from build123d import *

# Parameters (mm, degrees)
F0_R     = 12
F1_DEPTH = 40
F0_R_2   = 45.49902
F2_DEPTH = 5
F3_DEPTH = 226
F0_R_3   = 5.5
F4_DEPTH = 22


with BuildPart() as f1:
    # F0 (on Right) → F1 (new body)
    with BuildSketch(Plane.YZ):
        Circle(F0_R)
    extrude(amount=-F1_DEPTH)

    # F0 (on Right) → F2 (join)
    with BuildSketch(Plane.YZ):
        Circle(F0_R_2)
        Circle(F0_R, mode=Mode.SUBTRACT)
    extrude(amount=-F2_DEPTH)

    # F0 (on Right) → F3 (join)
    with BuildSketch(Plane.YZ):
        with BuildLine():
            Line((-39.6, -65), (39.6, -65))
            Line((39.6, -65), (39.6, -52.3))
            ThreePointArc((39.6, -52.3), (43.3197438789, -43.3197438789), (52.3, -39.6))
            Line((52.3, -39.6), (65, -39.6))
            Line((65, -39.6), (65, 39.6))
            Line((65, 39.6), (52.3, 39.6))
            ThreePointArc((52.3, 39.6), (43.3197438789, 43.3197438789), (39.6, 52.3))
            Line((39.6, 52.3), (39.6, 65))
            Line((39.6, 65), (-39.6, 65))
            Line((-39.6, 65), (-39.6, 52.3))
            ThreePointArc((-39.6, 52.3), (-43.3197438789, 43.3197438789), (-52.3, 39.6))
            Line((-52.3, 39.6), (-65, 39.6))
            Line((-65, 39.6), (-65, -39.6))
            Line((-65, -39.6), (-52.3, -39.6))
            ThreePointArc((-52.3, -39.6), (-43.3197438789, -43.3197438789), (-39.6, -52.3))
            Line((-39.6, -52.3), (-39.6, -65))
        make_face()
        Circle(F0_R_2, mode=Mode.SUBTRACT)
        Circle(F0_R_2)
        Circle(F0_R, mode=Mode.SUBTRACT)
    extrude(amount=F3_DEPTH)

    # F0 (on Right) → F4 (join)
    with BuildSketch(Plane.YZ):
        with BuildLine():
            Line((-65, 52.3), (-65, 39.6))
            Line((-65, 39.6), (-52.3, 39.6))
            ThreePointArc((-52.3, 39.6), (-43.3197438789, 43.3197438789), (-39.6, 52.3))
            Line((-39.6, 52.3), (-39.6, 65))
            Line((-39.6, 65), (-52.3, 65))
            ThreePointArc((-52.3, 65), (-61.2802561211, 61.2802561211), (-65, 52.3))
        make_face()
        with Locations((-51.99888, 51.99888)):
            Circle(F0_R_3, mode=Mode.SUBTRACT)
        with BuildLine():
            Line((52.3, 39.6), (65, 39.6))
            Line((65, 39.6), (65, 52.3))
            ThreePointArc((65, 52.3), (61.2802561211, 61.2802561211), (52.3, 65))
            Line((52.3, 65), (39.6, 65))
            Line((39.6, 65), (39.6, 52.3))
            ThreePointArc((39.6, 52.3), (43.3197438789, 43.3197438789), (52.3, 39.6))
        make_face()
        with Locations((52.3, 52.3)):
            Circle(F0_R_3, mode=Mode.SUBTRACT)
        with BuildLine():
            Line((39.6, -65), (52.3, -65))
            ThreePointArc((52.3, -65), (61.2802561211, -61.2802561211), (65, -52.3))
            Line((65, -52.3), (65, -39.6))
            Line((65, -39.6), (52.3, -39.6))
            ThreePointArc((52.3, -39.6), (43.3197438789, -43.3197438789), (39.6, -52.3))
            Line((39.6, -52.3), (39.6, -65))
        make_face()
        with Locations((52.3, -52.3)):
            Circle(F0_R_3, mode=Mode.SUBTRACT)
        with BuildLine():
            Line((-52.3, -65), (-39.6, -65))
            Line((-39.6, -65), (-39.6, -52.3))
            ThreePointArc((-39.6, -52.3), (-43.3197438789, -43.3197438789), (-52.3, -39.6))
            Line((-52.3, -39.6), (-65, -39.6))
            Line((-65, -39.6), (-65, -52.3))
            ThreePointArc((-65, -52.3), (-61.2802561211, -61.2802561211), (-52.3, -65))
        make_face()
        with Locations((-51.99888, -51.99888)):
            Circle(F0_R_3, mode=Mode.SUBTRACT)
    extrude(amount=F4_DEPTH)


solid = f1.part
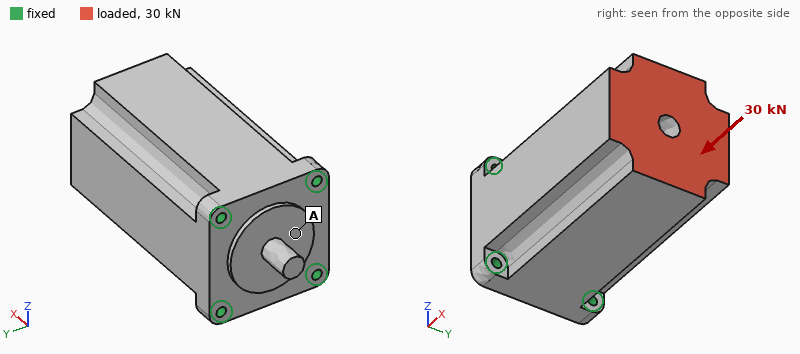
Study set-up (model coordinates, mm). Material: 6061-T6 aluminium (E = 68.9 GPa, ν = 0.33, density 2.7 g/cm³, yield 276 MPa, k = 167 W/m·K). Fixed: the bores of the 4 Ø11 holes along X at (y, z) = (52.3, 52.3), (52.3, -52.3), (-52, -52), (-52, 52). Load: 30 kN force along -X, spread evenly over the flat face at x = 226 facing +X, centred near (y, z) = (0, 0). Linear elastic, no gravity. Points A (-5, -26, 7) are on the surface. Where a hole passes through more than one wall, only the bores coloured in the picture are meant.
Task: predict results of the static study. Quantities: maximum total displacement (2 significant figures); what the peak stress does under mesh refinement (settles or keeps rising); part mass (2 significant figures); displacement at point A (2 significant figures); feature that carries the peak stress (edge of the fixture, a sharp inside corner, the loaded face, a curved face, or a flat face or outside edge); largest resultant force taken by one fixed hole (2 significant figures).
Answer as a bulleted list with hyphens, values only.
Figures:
- 14 µm
- keeps rising
- 8.8 kg
- 8.2 µm
- edge of the fixture
- 7.9 kN
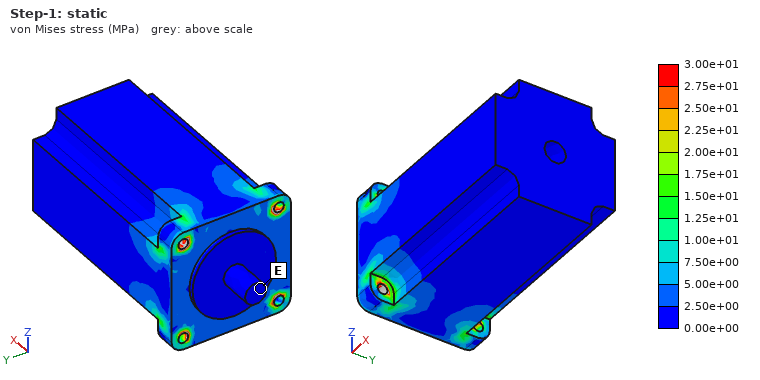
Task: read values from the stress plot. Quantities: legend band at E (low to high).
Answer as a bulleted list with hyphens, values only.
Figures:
- 0.00e+00 to 2.50e+00 MPa
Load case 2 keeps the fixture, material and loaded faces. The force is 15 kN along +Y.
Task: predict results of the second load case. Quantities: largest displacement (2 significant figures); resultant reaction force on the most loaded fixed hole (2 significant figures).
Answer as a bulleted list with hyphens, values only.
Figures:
- 0.12 mm
- 17 kN
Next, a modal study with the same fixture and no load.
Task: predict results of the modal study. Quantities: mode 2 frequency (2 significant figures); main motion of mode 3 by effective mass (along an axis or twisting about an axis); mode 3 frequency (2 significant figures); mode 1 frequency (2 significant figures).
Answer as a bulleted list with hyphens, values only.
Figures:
- 1100 Hz
- along X
- 3100 Hz
- 1100 Hz
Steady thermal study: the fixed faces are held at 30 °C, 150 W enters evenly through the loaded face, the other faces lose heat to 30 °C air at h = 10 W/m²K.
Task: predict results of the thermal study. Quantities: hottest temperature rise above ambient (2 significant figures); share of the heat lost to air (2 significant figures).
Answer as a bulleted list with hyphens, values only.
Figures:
- 17 K
- 9.1 %
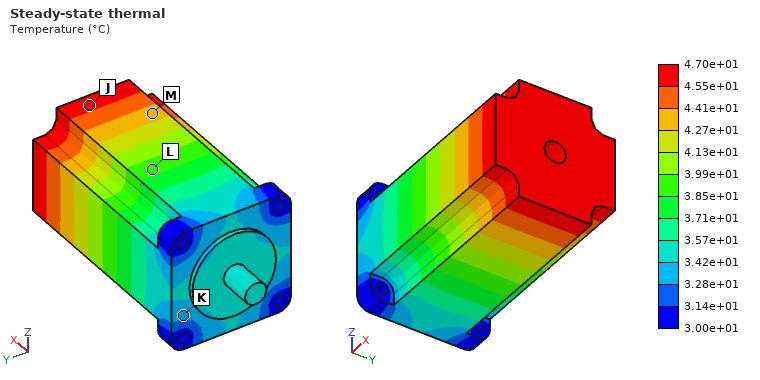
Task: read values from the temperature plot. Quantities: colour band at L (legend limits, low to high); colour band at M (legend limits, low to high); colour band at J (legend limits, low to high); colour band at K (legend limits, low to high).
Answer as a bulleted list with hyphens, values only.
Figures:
- 3.85e+01 to 3.99e+01 °C
- 4.27e+01 to 4.41e+01 °C
- 4.55e+01 to 4.70e+01 °C
- 3.28e+01 to 3.42e+01 °C
